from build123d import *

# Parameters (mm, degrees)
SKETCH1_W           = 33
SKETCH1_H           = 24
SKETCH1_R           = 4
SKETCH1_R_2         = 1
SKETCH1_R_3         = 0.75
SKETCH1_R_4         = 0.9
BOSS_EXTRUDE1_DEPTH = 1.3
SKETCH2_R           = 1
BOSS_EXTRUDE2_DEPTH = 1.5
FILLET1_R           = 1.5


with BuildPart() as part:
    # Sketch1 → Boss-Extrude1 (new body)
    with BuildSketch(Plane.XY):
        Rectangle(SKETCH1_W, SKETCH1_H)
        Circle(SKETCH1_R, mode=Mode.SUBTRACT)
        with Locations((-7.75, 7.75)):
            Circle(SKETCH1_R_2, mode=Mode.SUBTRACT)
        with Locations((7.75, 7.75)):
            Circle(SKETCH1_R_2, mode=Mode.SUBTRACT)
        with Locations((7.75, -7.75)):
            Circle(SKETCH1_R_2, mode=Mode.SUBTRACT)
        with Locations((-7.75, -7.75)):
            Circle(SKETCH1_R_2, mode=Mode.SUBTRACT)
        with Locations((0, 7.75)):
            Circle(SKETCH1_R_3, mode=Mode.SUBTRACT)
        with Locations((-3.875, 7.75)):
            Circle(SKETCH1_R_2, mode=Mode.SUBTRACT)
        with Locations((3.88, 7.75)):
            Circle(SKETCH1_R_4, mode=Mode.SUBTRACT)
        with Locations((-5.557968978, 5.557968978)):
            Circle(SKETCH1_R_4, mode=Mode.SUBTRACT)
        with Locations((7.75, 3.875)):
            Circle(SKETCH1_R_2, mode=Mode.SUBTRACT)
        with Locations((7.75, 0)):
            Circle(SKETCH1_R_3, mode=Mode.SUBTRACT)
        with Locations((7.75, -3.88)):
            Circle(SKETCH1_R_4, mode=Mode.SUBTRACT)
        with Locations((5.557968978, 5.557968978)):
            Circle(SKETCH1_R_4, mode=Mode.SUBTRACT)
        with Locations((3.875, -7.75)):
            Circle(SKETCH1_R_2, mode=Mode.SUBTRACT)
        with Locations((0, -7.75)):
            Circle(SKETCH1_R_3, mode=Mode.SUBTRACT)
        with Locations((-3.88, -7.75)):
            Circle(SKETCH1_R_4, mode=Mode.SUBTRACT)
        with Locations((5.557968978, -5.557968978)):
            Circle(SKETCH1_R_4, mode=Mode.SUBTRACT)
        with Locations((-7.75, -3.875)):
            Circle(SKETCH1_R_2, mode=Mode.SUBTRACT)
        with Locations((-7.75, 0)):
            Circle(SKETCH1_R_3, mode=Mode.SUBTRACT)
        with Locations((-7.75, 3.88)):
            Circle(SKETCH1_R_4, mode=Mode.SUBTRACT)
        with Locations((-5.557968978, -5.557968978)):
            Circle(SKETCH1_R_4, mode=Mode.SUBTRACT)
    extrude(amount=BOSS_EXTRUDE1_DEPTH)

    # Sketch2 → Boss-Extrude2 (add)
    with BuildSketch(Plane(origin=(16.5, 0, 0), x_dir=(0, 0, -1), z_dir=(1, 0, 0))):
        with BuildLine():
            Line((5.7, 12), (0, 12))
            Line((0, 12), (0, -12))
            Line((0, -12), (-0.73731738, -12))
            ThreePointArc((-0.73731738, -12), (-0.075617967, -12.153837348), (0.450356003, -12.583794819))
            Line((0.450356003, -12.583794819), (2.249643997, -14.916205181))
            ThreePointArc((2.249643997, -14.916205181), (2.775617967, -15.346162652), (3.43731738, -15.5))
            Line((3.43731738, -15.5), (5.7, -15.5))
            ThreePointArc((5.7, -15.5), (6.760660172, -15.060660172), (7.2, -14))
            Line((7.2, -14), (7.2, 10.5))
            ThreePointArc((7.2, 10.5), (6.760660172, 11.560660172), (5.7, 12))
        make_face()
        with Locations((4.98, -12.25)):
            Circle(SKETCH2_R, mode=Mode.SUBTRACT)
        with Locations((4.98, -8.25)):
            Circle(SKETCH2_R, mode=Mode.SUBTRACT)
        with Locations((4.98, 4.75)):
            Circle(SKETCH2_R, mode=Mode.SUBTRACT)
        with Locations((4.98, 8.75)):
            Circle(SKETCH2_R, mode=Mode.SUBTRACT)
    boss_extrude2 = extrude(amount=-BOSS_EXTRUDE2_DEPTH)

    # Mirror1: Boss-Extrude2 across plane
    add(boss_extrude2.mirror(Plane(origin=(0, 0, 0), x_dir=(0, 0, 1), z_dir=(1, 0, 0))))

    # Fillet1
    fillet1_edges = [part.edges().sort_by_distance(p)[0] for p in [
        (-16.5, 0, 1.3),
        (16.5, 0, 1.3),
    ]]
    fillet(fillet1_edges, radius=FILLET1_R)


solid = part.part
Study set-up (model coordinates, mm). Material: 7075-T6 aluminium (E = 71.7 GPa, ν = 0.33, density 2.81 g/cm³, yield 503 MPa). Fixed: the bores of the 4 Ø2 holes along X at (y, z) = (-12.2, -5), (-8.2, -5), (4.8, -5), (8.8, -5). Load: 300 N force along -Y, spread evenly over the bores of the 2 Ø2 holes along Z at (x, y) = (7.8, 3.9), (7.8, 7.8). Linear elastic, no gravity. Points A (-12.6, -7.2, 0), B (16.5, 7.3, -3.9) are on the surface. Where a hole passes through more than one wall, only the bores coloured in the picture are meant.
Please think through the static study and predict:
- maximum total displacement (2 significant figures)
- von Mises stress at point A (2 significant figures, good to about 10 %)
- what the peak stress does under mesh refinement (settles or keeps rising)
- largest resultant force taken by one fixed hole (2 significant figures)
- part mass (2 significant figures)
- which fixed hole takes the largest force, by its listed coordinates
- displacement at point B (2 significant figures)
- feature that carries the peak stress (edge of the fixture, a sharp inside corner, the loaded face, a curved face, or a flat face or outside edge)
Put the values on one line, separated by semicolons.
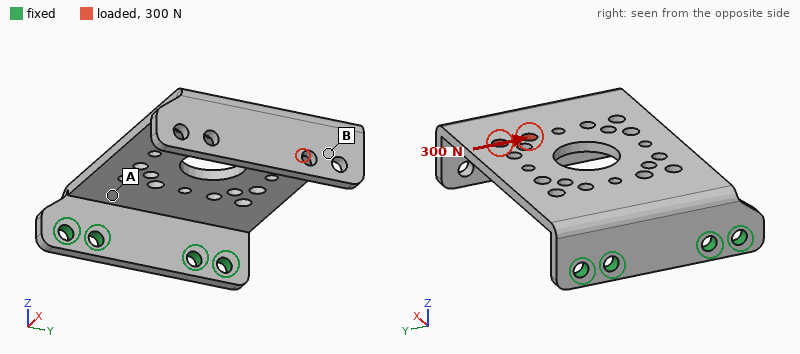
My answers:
0.42 mm; 120 MPa; keeps rising; 290 N; 4.0 g; (8.8, -5); 0.36 mm; edge of the fixture
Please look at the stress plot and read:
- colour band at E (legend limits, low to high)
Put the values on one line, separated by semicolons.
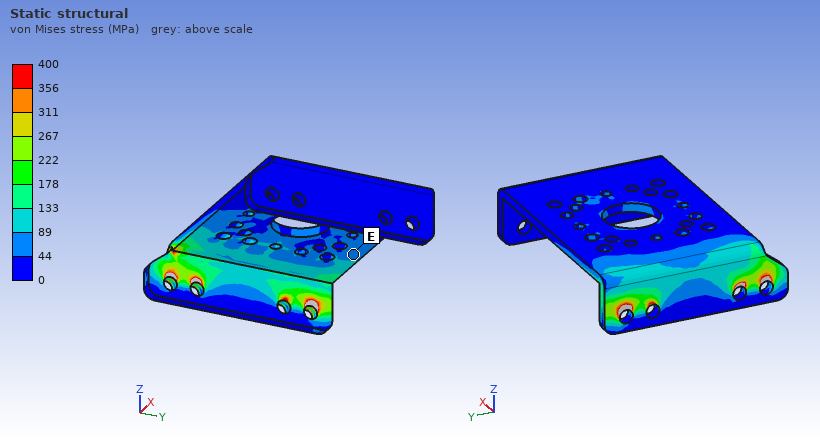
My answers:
44 to 89 MPa
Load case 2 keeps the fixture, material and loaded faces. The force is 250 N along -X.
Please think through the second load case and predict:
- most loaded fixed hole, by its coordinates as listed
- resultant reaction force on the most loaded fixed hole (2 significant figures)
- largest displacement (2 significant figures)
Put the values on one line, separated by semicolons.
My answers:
(8.8, -5); 130 N; 0.27 mm
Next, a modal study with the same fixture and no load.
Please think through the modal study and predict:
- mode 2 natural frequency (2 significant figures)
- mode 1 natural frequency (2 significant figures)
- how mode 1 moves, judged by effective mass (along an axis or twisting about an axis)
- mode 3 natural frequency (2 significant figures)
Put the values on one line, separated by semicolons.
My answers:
1800 Hz; 600 Hz; along Z; 3700 Hz
